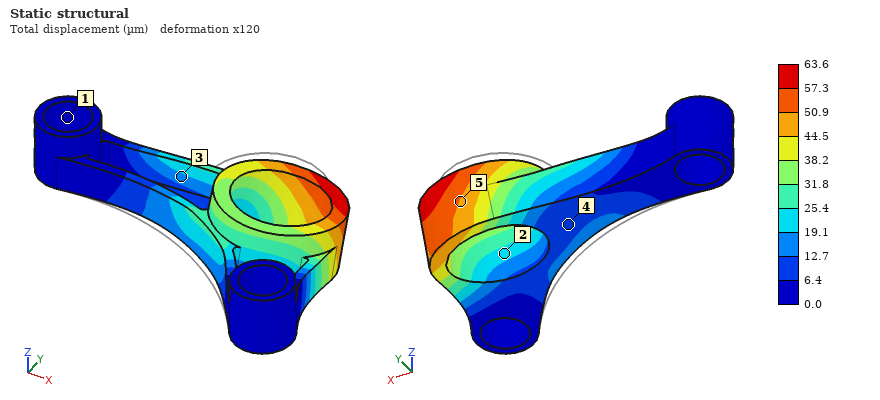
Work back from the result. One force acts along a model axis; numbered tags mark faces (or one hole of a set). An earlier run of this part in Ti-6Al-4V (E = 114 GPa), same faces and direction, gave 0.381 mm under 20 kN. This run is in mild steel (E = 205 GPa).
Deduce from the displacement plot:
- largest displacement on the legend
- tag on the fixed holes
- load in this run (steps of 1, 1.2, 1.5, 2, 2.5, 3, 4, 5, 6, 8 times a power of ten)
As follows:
63.6 µm
1
6 kN
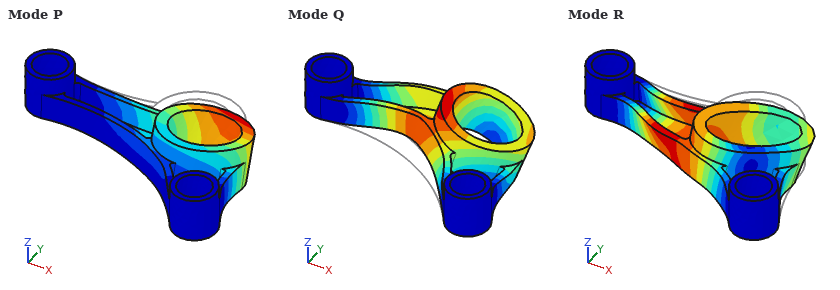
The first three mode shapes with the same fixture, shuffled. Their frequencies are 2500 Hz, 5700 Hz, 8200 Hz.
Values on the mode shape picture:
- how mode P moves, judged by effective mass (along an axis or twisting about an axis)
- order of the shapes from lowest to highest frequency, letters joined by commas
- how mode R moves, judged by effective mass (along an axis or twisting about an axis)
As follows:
along Z
P, Q, R
along Y
